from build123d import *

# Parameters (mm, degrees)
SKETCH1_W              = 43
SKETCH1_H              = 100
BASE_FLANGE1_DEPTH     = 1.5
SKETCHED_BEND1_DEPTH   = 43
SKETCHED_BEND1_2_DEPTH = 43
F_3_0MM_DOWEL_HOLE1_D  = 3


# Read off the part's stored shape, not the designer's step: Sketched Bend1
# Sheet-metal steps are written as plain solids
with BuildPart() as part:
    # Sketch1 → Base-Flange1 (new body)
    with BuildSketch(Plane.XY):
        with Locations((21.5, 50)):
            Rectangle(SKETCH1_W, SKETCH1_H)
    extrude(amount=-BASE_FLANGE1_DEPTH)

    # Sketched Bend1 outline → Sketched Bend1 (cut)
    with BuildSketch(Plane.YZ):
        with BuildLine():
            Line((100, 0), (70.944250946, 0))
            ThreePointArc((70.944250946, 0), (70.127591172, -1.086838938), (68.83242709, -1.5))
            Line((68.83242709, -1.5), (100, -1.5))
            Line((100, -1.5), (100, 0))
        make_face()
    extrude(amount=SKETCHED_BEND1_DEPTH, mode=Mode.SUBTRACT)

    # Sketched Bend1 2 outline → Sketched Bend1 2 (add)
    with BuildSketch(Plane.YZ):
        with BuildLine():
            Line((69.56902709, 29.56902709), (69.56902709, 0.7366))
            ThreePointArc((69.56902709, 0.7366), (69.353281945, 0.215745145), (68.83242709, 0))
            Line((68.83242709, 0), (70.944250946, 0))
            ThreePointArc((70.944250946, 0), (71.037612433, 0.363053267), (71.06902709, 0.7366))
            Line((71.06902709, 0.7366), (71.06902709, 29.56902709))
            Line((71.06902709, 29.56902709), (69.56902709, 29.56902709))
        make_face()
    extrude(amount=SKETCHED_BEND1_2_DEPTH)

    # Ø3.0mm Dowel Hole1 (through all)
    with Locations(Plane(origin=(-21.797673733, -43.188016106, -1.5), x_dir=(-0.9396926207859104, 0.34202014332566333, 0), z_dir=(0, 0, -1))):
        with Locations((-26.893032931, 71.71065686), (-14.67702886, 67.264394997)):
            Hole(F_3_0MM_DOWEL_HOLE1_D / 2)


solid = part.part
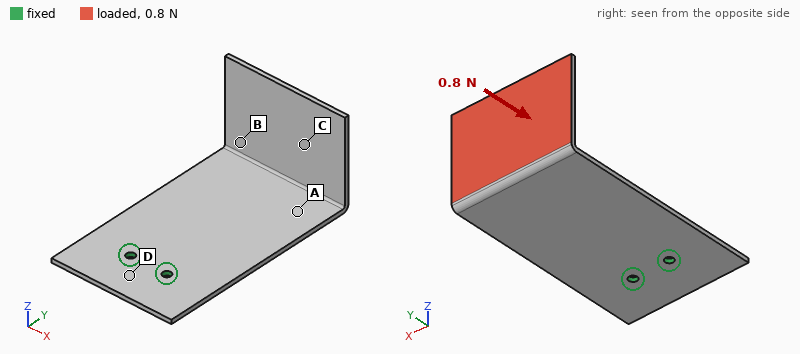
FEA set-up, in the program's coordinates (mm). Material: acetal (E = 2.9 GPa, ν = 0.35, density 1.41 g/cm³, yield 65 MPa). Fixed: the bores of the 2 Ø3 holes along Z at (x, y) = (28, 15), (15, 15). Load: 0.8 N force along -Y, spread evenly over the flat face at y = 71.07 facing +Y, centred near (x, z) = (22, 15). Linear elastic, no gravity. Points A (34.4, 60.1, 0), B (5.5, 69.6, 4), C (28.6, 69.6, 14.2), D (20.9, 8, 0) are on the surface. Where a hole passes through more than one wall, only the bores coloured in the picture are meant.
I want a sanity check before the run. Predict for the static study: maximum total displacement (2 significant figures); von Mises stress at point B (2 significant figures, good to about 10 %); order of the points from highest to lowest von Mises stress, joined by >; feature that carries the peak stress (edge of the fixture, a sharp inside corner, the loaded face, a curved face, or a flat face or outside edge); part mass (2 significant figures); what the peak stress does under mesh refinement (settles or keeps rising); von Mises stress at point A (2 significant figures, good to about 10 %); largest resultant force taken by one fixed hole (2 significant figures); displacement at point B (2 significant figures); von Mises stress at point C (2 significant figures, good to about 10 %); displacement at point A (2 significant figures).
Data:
0.85 mm
0.47 MPa
A > B > C > D
edge of the fixture
9.1 g
keeps rising
0.74 MPa
0.40 N
0.53 mm
0.18 MPa
0.36 mm
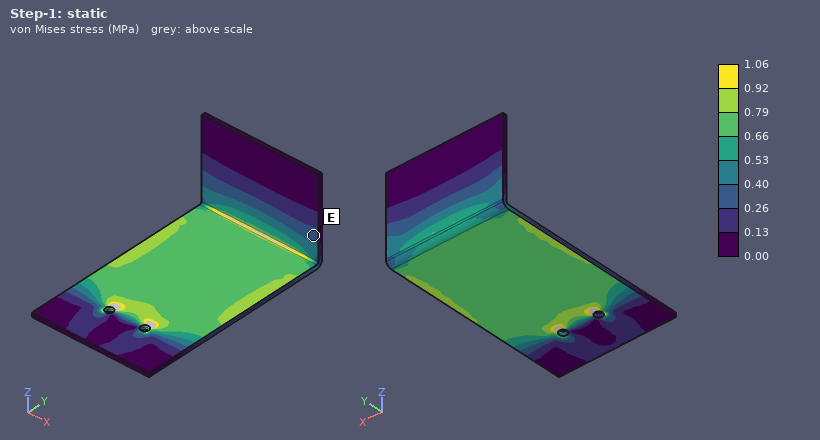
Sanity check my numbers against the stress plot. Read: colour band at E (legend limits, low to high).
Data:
0.26 to 0.40 MPa
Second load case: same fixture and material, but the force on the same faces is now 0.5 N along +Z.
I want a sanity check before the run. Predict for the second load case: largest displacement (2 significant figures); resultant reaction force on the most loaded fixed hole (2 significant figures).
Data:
1.0 mm
0.25 N
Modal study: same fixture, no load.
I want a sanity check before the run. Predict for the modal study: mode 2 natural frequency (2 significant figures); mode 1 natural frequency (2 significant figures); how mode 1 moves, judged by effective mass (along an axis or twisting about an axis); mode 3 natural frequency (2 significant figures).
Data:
140 Hz
60 Hz
along Z
230 Hz
